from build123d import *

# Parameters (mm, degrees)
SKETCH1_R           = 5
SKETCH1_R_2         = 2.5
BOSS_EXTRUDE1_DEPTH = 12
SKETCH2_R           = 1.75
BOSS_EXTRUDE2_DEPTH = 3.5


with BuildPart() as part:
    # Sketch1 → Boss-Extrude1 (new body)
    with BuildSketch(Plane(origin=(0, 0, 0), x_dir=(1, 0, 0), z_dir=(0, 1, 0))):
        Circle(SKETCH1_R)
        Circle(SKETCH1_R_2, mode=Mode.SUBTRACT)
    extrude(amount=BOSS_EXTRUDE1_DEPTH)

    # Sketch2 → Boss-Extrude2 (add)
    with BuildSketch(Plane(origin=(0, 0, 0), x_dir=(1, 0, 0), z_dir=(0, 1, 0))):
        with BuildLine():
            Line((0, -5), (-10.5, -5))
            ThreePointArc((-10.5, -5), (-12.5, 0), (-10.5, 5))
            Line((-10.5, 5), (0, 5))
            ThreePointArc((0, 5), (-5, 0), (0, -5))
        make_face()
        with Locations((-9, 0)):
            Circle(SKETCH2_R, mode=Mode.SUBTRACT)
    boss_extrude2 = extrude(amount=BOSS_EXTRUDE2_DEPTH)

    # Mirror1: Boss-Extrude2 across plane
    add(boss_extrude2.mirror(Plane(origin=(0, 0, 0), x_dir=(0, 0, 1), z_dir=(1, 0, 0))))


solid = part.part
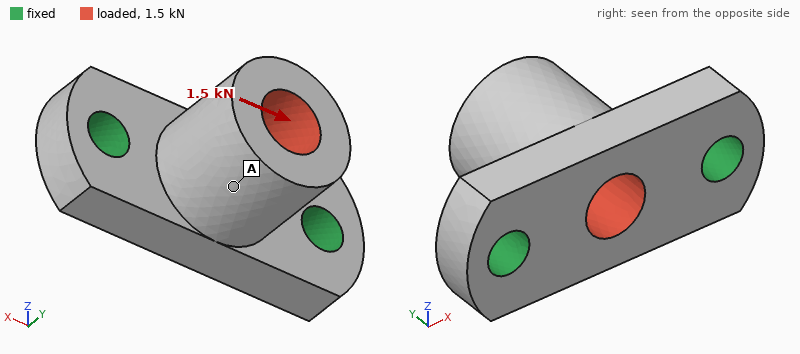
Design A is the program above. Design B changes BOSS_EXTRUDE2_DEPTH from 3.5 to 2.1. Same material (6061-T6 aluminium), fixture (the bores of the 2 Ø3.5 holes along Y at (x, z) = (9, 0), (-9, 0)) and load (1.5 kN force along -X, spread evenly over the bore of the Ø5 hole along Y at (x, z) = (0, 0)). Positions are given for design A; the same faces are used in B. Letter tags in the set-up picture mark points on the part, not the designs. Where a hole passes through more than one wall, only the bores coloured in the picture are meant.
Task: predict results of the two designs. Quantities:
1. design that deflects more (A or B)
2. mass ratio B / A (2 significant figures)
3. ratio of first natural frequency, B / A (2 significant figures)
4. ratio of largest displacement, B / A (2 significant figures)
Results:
B
0.84
0.56
2.2
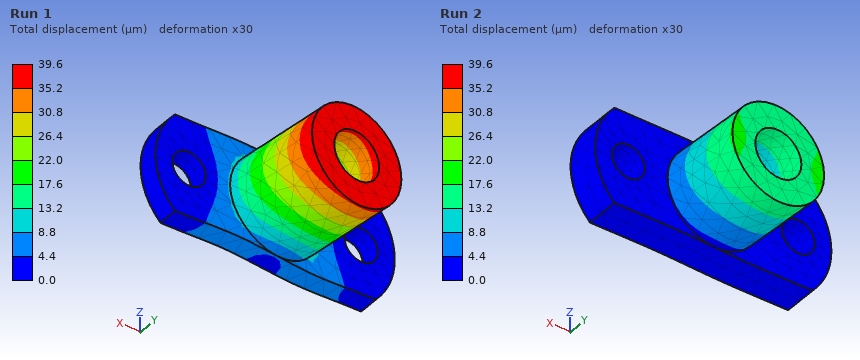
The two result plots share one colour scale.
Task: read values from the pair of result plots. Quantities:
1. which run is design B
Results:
Run 1
